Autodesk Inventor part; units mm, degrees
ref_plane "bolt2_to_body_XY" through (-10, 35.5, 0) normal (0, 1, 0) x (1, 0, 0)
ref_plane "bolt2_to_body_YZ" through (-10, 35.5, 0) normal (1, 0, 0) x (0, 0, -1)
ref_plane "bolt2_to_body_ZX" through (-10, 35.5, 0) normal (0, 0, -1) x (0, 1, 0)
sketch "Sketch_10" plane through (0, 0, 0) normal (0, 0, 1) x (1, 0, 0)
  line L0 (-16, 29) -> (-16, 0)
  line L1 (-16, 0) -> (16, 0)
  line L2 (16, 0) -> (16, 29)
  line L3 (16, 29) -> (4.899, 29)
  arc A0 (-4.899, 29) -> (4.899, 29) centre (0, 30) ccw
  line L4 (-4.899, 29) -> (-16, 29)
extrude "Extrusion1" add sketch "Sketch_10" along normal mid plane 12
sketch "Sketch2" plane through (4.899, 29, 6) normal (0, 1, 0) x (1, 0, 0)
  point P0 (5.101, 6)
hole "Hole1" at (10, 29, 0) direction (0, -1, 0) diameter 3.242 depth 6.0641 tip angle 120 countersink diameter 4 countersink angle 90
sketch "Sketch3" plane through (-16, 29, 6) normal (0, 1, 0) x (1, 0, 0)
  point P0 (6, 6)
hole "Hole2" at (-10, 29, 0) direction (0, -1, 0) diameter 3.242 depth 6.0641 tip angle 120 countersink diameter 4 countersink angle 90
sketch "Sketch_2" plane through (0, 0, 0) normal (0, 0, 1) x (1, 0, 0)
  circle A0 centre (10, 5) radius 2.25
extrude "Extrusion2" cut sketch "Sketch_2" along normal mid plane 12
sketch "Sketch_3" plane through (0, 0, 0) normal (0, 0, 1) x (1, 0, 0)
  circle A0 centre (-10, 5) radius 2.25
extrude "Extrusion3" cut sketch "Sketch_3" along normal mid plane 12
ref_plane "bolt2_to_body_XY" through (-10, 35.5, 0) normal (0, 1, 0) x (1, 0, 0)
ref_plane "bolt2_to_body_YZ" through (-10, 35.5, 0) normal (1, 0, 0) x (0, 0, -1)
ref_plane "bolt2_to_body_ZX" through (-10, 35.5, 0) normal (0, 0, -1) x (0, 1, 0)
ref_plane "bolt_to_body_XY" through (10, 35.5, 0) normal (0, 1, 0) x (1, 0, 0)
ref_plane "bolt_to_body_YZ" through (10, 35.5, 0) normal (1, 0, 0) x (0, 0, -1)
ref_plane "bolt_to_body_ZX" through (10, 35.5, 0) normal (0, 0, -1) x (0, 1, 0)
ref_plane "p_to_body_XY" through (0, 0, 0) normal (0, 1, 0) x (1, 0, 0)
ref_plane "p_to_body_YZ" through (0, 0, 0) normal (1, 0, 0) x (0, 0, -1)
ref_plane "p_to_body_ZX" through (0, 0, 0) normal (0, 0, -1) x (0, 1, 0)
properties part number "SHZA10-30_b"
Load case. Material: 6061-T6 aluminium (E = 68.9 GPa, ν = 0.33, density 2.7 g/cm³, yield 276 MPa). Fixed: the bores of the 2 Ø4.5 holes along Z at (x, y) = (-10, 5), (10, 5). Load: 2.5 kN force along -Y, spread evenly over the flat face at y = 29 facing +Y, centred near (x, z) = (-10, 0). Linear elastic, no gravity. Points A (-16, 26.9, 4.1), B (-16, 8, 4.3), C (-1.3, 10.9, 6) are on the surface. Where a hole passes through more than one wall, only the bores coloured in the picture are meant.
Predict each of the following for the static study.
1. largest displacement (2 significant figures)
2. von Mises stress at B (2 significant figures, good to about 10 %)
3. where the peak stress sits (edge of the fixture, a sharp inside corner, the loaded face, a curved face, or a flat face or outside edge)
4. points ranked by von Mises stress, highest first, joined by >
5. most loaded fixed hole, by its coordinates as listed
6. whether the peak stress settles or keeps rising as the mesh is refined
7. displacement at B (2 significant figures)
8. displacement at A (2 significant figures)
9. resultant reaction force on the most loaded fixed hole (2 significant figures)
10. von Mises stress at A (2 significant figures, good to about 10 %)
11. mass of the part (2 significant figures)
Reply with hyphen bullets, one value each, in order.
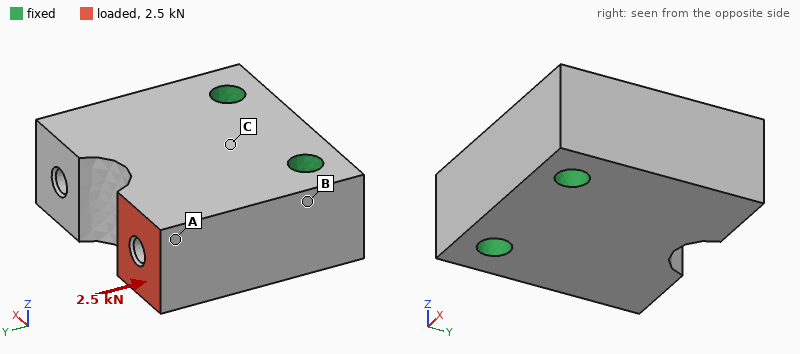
- 9.5 µm
- 11 MPa
- edge of the fixture
- A > B > C
- (-10, 5)
- keeps rising
- 1.8 µm
- 8.5 µm
- 2.4 kN
- 21 MPa
- 28 g
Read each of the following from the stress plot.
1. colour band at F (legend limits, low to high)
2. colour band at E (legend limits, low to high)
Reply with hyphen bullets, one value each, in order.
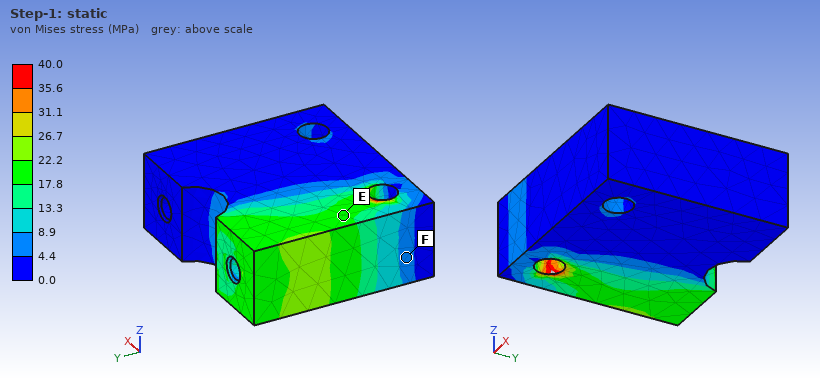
- 4.4 to 8.9 MPa
- 17.8 to 22.2 MPa
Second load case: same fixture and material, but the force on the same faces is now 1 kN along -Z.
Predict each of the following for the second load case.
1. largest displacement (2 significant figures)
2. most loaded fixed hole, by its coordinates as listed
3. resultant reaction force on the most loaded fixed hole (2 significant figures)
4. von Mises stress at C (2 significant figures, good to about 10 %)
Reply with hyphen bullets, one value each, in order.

- 32 µm
- (-10, 5)
- 880 N
- 18 MPa
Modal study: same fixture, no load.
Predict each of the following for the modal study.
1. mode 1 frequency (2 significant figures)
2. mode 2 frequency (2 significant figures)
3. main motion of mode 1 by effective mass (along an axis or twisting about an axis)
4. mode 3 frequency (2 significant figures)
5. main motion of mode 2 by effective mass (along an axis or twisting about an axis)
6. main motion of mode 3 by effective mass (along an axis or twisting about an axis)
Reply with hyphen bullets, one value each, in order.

- 15 kHz
- 24 kHz
- along Z
- 25 kHz
- twisting about Y
- along X
